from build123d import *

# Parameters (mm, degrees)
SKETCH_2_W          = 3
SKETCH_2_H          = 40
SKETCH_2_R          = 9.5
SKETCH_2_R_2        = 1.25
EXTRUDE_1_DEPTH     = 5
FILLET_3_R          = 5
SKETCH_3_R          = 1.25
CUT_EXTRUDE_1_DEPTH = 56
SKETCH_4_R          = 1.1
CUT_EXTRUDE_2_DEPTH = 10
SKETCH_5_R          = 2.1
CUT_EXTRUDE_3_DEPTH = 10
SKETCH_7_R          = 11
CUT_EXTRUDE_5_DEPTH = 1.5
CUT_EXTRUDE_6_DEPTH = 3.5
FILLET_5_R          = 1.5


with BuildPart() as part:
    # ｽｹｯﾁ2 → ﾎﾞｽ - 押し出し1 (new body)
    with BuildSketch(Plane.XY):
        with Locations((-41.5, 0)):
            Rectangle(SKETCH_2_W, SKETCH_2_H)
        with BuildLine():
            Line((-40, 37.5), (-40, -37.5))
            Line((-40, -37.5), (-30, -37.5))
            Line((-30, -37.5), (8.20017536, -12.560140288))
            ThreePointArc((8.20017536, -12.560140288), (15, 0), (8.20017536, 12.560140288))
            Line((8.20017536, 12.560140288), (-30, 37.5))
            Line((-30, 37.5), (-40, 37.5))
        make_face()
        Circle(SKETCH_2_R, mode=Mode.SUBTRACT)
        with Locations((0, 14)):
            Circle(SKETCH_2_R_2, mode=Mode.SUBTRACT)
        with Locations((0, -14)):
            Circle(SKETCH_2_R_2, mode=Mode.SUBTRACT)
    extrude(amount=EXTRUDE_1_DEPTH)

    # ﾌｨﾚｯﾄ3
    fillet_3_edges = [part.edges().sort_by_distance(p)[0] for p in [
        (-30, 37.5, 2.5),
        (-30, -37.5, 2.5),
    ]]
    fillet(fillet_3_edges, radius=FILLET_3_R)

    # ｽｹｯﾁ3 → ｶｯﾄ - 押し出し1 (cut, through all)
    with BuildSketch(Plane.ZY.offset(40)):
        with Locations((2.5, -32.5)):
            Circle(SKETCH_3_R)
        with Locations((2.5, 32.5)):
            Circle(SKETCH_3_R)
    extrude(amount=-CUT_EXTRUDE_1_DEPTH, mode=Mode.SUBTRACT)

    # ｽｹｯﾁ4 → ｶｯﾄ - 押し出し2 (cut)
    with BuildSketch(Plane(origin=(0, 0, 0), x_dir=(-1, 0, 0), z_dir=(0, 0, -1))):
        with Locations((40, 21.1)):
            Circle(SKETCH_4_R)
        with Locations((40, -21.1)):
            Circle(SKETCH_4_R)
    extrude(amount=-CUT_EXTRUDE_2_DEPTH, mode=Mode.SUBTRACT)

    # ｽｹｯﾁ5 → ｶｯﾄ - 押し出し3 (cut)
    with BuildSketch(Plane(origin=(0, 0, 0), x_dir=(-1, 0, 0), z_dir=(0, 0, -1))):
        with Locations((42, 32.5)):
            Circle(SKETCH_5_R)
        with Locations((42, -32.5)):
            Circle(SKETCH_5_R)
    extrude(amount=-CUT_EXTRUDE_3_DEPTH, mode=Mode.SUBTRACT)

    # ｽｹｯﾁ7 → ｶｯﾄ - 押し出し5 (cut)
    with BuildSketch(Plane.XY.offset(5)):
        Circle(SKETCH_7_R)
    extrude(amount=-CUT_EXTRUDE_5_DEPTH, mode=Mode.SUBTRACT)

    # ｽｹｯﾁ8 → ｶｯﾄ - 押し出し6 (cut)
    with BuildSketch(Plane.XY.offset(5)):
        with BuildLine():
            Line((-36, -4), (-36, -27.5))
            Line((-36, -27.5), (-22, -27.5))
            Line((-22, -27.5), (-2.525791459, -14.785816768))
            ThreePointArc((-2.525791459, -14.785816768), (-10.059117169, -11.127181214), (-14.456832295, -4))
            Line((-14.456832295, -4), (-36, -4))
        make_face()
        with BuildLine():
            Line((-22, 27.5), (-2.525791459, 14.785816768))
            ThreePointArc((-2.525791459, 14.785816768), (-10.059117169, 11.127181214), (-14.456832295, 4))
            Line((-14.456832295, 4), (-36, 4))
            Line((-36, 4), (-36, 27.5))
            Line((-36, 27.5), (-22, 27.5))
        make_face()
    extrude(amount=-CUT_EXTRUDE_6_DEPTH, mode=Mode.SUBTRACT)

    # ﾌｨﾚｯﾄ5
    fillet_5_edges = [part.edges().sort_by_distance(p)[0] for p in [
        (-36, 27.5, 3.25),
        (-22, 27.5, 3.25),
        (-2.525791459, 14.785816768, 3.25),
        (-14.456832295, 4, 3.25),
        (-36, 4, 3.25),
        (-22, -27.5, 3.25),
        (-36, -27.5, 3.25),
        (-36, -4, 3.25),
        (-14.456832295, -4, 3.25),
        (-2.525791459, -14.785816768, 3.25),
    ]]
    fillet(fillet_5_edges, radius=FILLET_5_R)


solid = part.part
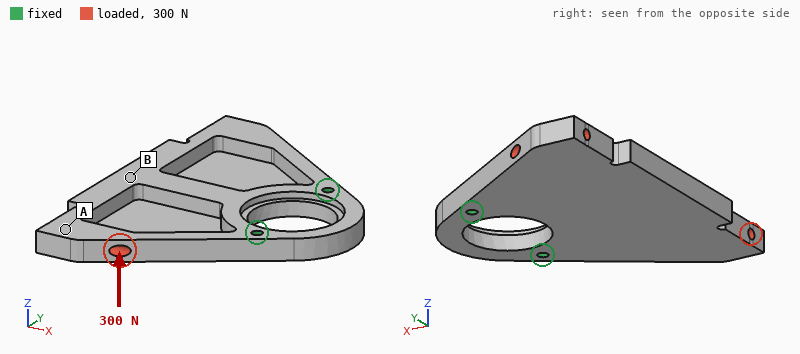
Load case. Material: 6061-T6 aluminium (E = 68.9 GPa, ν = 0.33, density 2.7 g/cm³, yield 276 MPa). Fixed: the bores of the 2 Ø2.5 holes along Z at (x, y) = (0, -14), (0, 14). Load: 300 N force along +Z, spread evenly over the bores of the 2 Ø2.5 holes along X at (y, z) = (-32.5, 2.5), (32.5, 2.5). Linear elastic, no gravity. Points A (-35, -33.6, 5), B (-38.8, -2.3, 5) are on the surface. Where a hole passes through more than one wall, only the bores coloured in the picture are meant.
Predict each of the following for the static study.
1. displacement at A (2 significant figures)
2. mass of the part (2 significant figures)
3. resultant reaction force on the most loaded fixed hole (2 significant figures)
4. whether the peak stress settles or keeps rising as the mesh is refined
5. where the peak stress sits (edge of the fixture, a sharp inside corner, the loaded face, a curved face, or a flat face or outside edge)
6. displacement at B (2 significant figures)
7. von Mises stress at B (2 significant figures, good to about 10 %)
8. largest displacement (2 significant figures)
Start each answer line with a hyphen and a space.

- 0.36 mm
- 24 g
- 170 N
- keeps rising
- edge of the fixture
- 0.31 mm
- 36 MPa
- 0.43 mm
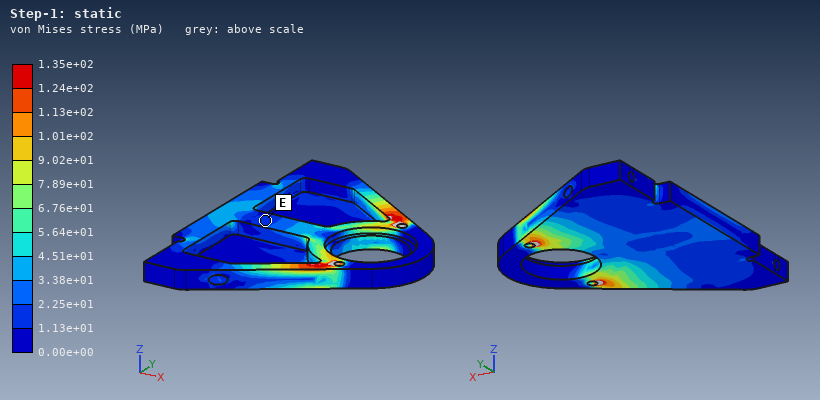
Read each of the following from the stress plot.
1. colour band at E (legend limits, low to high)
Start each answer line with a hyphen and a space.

- 1.13e+01 to 2.25e+01 MPa
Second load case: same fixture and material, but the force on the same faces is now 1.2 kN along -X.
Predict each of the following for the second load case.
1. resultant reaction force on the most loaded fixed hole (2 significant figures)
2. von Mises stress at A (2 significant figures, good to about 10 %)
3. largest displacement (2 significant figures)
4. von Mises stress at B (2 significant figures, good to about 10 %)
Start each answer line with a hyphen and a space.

- 630 N
- 7.4 MPa
- 42 µm
- 3.3 MPa
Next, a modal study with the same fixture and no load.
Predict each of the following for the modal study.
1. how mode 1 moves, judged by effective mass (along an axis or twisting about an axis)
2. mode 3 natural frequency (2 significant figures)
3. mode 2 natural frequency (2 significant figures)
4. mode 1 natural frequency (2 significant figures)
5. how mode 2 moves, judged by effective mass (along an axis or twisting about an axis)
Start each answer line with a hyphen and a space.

- along Z
- 4600 Hz
- 2000 Hz
- 1300 Hz
- twisting about X
